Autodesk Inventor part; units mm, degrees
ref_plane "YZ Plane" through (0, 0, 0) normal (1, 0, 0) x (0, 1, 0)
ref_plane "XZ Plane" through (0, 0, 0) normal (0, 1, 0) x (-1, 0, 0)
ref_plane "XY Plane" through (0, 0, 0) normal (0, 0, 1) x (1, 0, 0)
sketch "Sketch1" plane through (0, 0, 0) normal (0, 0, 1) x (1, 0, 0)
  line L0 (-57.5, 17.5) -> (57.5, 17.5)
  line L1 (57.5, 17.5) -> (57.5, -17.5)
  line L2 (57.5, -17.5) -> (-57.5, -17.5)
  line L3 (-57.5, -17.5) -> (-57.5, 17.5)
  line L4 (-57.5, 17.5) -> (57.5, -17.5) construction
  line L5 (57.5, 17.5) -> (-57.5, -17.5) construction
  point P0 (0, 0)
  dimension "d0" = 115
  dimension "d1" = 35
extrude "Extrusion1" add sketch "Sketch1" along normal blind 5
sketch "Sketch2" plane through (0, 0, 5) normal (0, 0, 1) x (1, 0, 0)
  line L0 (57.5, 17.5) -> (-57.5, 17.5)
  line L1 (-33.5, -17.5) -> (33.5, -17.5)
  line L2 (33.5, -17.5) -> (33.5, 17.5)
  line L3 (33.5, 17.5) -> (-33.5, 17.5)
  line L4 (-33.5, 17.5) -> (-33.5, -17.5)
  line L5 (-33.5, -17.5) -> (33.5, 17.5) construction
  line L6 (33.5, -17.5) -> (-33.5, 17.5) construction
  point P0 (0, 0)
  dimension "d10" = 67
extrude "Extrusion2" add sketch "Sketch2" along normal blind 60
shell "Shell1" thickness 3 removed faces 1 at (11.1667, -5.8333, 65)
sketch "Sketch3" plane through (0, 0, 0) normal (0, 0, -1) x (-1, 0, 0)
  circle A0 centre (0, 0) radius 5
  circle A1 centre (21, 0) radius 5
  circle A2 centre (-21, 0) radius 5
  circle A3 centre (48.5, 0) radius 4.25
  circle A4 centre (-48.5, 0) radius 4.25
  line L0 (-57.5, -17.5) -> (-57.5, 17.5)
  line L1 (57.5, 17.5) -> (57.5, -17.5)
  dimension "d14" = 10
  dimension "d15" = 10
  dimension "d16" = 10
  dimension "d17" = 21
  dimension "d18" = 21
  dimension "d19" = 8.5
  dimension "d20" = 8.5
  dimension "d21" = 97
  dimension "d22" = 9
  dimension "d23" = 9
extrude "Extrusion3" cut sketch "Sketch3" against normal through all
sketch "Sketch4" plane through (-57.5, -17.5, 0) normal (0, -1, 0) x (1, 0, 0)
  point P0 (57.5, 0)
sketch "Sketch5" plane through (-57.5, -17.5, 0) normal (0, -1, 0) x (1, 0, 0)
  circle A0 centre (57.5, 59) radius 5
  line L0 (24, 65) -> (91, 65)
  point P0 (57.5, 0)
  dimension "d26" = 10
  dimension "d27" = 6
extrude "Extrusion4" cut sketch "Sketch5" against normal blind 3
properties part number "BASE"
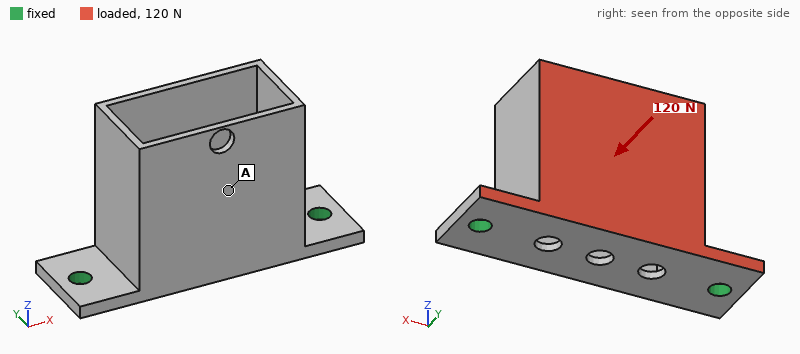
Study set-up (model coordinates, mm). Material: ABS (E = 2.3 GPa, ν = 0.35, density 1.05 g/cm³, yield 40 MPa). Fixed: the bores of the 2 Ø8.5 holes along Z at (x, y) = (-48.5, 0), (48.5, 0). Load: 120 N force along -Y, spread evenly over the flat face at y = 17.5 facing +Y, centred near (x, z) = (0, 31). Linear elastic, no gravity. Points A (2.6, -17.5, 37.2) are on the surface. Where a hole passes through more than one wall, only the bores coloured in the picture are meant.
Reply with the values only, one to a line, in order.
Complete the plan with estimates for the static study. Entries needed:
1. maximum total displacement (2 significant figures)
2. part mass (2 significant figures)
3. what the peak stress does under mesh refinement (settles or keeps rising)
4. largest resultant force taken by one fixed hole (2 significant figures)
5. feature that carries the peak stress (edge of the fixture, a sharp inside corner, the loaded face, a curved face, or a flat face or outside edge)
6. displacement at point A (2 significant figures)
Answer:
1.4 mm
52 g
keeps rising
60 N
edge of the fixture
0.56 mm
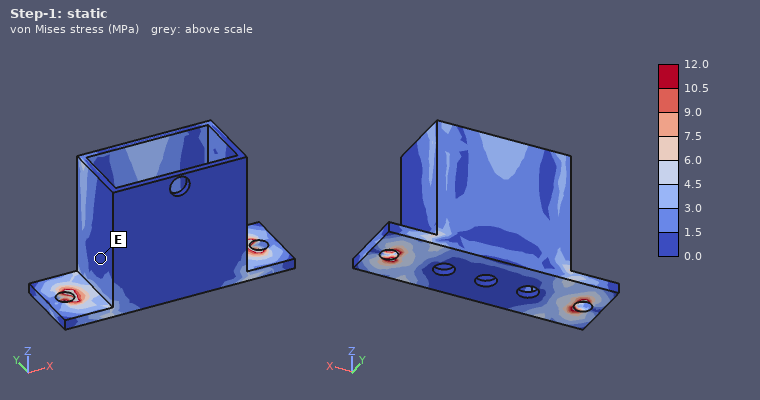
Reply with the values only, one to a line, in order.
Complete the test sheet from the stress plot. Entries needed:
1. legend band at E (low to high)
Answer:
0.0 to 1.5 MPa
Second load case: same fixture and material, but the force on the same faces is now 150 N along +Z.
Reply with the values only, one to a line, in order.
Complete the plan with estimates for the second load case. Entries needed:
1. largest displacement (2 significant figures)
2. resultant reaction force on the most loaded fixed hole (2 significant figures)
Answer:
0.80 mm
77 N
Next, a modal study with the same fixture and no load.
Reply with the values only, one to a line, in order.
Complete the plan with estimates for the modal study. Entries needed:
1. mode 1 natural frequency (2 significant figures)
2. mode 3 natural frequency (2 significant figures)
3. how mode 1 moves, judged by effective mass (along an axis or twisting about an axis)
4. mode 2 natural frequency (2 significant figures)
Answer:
310 Hz
860 Hz
along Y
700 Hz
